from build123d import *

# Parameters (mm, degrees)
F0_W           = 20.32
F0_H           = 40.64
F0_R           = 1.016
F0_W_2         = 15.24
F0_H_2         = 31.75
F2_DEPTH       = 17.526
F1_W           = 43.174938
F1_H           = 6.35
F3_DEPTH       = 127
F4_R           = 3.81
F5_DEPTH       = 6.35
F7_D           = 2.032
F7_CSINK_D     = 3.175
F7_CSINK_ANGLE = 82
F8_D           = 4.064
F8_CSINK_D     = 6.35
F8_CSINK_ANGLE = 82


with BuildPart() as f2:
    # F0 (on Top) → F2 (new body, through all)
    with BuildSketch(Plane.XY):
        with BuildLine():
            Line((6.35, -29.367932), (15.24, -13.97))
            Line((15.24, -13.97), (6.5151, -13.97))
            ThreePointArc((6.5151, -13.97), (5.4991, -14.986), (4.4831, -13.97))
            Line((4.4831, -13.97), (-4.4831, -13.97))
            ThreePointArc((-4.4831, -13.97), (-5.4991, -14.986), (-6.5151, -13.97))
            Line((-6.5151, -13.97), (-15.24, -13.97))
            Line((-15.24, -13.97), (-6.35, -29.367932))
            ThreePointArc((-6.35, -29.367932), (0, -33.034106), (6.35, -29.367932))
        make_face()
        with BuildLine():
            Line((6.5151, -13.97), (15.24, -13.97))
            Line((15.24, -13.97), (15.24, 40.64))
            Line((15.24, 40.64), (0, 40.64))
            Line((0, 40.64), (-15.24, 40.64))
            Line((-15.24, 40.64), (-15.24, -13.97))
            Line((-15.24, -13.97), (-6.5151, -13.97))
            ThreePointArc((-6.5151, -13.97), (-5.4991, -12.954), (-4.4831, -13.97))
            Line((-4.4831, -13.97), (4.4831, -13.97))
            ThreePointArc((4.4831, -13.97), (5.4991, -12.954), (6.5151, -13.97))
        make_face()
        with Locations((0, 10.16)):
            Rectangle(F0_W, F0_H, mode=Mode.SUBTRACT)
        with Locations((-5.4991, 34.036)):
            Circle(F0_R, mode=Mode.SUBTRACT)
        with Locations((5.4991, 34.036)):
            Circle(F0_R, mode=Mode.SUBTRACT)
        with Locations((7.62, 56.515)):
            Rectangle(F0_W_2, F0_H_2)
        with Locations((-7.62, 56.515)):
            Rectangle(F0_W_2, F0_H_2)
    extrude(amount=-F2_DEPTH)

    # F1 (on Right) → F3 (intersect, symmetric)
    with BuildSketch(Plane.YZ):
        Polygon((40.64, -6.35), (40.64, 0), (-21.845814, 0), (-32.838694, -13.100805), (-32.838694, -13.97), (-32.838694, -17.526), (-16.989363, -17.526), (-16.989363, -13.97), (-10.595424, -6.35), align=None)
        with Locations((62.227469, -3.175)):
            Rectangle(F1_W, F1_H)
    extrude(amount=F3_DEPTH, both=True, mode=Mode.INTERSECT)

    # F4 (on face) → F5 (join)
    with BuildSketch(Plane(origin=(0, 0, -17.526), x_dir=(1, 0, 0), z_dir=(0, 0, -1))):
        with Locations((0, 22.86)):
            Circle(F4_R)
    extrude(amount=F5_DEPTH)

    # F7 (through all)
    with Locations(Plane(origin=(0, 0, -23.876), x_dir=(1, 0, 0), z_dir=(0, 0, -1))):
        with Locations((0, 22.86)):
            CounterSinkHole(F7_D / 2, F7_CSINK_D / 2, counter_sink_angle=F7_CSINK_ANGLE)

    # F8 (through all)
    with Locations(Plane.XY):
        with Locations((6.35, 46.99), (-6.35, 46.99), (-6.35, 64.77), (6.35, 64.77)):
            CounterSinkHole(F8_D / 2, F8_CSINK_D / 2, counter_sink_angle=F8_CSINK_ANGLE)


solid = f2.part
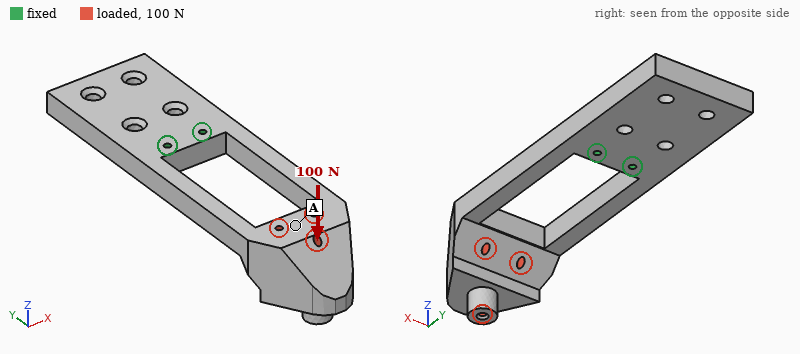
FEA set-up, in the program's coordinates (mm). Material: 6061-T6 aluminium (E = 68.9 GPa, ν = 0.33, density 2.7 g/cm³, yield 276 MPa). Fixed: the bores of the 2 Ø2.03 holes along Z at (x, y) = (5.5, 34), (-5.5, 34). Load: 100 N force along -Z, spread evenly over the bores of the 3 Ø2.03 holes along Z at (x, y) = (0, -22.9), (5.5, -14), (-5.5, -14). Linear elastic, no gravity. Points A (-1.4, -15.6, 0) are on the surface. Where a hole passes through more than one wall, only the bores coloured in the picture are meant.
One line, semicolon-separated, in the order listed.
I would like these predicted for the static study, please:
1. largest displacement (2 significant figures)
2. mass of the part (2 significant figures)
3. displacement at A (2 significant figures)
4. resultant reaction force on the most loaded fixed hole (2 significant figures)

0.54 mm; 44 g; 0.35 mm; 50 N
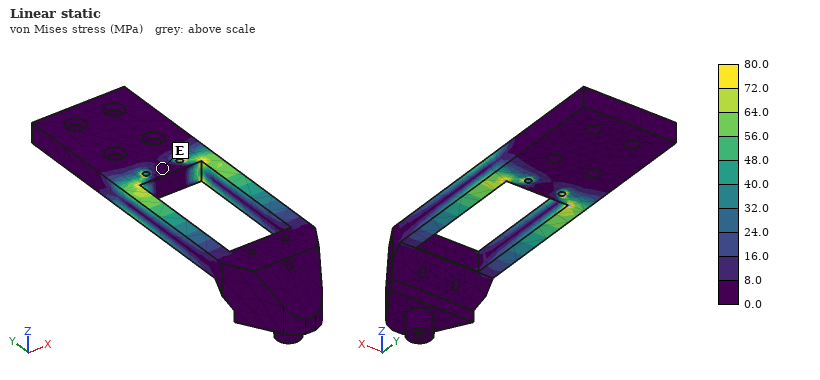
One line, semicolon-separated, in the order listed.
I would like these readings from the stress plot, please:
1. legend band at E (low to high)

0.0 to 8.0 MPa
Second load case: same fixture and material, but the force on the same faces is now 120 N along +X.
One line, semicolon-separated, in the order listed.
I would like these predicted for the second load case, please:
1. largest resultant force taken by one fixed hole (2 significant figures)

490 N
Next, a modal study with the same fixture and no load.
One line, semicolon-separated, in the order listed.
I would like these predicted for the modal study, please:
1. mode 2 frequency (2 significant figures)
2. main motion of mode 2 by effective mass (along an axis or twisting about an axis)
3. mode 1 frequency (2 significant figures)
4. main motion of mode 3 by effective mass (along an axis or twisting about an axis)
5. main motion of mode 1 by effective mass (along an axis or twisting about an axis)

1100 Hz; along X; 580 Hz; twisting about Y; along Z
